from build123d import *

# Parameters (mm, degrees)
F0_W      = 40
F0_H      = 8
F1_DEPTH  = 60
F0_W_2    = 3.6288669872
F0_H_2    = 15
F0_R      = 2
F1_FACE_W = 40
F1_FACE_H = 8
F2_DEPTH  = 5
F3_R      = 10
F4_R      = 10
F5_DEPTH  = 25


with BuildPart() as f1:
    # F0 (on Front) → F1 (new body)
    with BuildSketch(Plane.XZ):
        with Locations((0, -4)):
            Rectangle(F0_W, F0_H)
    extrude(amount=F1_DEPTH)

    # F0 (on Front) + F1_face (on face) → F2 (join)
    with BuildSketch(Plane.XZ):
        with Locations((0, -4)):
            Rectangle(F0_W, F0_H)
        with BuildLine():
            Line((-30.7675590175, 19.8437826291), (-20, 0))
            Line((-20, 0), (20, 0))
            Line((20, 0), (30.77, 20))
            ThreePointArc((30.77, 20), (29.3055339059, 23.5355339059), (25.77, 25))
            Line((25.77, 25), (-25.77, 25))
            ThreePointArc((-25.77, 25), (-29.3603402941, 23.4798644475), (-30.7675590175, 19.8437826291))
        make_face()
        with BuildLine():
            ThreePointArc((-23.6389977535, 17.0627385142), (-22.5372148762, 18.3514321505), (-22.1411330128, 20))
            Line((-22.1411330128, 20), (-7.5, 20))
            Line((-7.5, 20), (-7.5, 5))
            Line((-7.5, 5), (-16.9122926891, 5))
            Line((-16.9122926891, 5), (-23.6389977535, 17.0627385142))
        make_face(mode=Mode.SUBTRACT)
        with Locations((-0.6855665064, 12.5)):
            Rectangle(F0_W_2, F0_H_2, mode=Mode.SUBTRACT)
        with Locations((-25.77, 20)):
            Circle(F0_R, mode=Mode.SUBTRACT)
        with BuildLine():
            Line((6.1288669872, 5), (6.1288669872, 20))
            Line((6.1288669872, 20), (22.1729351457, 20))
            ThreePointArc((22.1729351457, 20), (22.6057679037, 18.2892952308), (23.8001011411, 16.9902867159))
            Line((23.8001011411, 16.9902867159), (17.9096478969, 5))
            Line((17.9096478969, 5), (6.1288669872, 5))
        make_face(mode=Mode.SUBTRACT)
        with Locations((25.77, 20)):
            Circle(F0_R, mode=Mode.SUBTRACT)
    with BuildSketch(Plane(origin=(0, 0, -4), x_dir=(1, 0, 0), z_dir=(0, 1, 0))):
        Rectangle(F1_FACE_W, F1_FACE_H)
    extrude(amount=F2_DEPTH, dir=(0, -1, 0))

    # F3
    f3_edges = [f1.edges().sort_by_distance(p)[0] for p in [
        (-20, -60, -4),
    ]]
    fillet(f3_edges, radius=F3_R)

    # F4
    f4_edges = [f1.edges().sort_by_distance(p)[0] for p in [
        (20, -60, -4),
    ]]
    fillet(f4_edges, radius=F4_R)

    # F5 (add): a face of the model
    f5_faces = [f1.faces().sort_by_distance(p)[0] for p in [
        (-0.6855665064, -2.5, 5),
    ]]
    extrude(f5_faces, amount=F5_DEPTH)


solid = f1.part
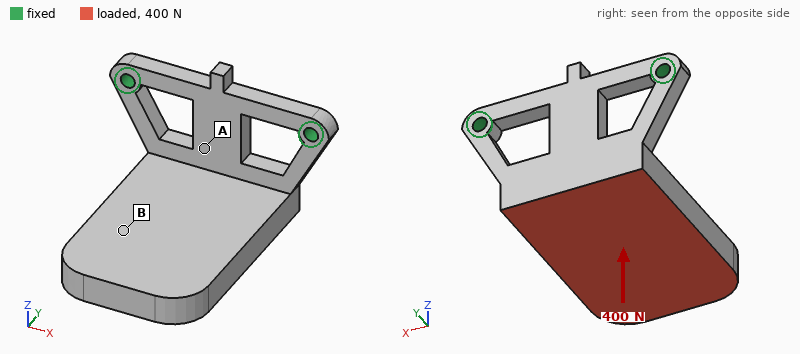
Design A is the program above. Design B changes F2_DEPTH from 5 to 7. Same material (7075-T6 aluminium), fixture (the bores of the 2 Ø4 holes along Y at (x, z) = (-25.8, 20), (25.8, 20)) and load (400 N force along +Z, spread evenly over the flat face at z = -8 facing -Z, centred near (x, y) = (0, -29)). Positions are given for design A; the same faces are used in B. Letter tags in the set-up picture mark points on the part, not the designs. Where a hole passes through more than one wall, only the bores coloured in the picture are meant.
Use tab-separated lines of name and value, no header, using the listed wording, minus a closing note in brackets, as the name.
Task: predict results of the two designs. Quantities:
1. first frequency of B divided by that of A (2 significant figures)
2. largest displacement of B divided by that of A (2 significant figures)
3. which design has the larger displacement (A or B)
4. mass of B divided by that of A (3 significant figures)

first frequency of B divided by that of A	1.6
largest displacement of B divided by that of A	0.41
which design has the larger displacement	A
mass of B divided by that of A	1.08
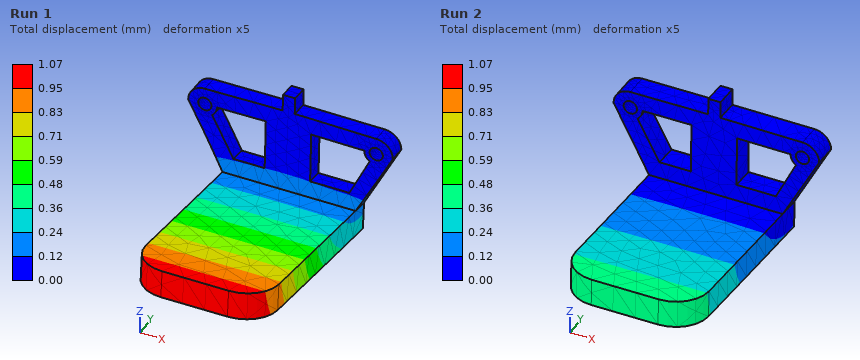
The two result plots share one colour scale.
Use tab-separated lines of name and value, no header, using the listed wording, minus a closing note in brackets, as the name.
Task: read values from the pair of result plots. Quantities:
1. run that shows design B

run that shows design B	Run 2
